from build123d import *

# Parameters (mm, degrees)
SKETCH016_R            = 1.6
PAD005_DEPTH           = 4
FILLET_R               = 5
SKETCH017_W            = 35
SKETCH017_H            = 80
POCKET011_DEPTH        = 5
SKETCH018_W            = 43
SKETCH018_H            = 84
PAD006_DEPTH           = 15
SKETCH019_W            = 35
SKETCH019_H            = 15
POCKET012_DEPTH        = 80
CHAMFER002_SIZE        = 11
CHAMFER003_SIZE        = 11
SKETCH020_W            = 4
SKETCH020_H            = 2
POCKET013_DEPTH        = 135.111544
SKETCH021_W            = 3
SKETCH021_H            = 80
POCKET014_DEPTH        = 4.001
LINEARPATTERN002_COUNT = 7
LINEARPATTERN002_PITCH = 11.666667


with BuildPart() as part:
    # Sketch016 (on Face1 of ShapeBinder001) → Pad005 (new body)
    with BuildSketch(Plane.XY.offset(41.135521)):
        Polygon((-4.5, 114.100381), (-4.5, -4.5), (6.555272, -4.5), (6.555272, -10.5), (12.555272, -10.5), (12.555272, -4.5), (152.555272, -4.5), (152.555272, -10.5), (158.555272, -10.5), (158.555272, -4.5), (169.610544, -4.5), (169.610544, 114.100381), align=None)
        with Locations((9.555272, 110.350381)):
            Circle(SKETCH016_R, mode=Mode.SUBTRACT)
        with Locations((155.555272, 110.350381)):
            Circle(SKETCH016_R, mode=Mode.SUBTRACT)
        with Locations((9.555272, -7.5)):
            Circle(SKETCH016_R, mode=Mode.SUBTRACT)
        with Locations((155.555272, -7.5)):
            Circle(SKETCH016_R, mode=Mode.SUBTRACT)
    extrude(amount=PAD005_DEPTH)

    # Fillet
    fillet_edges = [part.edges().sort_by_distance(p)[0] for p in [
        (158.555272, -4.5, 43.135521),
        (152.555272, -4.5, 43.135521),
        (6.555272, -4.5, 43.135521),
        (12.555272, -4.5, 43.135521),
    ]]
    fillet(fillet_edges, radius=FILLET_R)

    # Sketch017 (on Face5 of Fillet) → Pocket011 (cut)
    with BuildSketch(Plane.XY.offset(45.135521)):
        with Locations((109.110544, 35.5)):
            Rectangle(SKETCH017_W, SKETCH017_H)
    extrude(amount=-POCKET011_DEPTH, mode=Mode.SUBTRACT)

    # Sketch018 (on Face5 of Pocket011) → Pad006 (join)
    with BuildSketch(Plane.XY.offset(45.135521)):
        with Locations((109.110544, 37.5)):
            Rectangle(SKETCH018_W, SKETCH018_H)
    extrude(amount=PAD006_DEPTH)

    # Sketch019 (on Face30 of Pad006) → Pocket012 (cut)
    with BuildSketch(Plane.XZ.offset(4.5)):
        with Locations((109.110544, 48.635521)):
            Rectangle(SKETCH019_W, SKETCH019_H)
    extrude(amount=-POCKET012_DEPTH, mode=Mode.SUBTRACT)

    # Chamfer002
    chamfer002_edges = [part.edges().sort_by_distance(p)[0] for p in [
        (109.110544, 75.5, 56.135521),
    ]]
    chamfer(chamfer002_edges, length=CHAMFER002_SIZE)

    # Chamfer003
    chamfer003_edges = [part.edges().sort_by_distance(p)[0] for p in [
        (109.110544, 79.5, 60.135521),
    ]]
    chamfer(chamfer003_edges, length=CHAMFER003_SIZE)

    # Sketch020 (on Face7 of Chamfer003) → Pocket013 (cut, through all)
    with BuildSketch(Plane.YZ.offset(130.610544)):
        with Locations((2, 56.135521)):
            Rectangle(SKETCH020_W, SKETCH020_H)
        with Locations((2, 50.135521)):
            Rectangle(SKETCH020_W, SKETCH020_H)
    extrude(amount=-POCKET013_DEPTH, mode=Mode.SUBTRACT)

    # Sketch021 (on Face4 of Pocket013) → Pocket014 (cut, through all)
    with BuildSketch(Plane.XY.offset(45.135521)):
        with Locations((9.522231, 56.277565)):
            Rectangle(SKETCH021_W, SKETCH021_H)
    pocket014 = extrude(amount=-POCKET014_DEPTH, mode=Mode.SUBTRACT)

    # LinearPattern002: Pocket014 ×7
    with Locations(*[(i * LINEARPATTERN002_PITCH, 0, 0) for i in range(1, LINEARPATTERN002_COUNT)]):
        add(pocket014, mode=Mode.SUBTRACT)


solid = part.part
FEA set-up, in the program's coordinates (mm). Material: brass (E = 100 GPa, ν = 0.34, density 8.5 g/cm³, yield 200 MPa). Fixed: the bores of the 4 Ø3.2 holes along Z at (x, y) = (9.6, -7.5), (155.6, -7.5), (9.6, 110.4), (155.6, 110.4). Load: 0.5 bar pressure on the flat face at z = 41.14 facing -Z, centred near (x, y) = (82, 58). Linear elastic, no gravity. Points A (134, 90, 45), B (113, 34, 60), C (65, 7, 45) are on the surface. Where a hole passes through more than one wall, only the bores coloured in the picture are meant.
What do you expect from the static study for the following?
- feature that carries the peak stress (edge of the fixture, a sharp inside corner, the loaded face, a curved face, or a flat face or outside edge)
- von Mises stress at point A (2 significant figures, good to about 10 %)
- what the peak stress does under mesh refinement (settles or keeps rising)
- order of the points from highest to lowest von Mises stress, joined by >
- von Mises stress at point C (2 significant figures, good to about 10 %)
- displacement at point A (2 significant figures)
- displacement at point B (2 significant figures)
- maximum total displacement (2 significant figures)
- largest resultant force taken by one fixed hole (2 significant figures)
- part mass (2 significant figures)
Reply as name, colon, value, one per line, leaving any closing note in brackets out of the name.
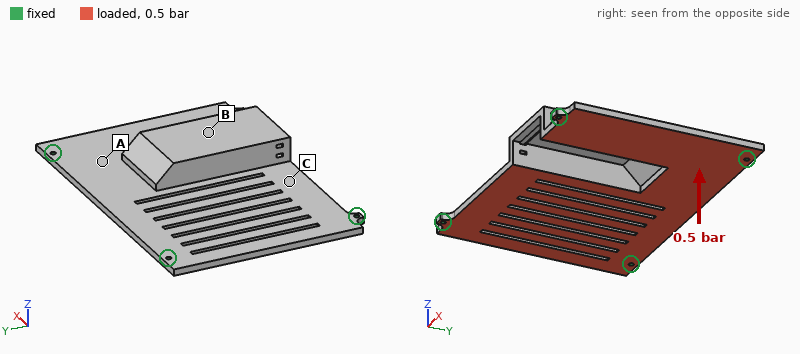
feature that carries the peak stress: edge of the fixture
von Mises stress at point A: 13 MPa
what the peak stress does under mesh refinement: keeps rising
order of the points from highest to lowest von Mises stress, joined by >: C > A > B
von Mises stress at point C: 37 MPa
displacement at point A: 0.091 mm
displacement at point B: 0.17 mm
maximum total displacement: 0.32 mm
largest resultant force taken by one fixed hole: 240 N
part mass: 740 g
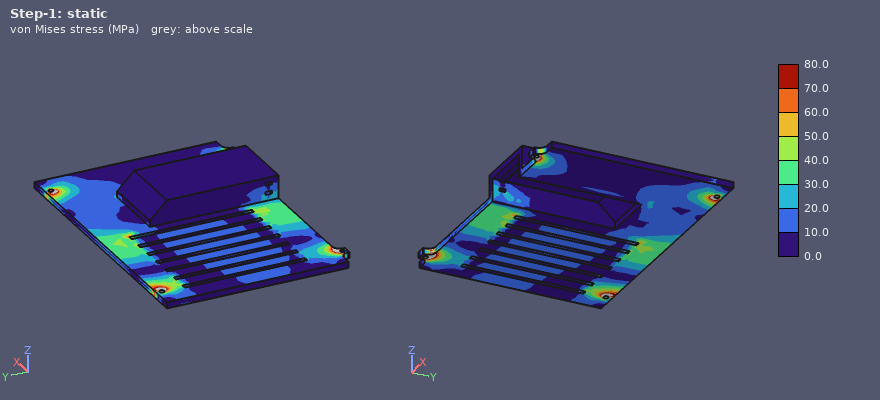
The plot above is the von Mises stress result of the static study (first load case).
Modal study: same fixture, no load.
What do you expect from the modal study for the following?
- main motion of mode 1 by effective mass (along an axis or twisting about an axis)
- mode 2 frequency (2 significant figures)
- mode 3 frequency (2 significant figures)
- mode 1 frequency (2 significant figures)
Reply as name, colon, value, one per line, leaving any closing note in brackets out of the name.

main motion of mode 1 by effective mass: along Z
mode 2 frequency: 820 Hz
mode 3 frequency: 830 Hz
mode 1 frequency: 340 Hz
